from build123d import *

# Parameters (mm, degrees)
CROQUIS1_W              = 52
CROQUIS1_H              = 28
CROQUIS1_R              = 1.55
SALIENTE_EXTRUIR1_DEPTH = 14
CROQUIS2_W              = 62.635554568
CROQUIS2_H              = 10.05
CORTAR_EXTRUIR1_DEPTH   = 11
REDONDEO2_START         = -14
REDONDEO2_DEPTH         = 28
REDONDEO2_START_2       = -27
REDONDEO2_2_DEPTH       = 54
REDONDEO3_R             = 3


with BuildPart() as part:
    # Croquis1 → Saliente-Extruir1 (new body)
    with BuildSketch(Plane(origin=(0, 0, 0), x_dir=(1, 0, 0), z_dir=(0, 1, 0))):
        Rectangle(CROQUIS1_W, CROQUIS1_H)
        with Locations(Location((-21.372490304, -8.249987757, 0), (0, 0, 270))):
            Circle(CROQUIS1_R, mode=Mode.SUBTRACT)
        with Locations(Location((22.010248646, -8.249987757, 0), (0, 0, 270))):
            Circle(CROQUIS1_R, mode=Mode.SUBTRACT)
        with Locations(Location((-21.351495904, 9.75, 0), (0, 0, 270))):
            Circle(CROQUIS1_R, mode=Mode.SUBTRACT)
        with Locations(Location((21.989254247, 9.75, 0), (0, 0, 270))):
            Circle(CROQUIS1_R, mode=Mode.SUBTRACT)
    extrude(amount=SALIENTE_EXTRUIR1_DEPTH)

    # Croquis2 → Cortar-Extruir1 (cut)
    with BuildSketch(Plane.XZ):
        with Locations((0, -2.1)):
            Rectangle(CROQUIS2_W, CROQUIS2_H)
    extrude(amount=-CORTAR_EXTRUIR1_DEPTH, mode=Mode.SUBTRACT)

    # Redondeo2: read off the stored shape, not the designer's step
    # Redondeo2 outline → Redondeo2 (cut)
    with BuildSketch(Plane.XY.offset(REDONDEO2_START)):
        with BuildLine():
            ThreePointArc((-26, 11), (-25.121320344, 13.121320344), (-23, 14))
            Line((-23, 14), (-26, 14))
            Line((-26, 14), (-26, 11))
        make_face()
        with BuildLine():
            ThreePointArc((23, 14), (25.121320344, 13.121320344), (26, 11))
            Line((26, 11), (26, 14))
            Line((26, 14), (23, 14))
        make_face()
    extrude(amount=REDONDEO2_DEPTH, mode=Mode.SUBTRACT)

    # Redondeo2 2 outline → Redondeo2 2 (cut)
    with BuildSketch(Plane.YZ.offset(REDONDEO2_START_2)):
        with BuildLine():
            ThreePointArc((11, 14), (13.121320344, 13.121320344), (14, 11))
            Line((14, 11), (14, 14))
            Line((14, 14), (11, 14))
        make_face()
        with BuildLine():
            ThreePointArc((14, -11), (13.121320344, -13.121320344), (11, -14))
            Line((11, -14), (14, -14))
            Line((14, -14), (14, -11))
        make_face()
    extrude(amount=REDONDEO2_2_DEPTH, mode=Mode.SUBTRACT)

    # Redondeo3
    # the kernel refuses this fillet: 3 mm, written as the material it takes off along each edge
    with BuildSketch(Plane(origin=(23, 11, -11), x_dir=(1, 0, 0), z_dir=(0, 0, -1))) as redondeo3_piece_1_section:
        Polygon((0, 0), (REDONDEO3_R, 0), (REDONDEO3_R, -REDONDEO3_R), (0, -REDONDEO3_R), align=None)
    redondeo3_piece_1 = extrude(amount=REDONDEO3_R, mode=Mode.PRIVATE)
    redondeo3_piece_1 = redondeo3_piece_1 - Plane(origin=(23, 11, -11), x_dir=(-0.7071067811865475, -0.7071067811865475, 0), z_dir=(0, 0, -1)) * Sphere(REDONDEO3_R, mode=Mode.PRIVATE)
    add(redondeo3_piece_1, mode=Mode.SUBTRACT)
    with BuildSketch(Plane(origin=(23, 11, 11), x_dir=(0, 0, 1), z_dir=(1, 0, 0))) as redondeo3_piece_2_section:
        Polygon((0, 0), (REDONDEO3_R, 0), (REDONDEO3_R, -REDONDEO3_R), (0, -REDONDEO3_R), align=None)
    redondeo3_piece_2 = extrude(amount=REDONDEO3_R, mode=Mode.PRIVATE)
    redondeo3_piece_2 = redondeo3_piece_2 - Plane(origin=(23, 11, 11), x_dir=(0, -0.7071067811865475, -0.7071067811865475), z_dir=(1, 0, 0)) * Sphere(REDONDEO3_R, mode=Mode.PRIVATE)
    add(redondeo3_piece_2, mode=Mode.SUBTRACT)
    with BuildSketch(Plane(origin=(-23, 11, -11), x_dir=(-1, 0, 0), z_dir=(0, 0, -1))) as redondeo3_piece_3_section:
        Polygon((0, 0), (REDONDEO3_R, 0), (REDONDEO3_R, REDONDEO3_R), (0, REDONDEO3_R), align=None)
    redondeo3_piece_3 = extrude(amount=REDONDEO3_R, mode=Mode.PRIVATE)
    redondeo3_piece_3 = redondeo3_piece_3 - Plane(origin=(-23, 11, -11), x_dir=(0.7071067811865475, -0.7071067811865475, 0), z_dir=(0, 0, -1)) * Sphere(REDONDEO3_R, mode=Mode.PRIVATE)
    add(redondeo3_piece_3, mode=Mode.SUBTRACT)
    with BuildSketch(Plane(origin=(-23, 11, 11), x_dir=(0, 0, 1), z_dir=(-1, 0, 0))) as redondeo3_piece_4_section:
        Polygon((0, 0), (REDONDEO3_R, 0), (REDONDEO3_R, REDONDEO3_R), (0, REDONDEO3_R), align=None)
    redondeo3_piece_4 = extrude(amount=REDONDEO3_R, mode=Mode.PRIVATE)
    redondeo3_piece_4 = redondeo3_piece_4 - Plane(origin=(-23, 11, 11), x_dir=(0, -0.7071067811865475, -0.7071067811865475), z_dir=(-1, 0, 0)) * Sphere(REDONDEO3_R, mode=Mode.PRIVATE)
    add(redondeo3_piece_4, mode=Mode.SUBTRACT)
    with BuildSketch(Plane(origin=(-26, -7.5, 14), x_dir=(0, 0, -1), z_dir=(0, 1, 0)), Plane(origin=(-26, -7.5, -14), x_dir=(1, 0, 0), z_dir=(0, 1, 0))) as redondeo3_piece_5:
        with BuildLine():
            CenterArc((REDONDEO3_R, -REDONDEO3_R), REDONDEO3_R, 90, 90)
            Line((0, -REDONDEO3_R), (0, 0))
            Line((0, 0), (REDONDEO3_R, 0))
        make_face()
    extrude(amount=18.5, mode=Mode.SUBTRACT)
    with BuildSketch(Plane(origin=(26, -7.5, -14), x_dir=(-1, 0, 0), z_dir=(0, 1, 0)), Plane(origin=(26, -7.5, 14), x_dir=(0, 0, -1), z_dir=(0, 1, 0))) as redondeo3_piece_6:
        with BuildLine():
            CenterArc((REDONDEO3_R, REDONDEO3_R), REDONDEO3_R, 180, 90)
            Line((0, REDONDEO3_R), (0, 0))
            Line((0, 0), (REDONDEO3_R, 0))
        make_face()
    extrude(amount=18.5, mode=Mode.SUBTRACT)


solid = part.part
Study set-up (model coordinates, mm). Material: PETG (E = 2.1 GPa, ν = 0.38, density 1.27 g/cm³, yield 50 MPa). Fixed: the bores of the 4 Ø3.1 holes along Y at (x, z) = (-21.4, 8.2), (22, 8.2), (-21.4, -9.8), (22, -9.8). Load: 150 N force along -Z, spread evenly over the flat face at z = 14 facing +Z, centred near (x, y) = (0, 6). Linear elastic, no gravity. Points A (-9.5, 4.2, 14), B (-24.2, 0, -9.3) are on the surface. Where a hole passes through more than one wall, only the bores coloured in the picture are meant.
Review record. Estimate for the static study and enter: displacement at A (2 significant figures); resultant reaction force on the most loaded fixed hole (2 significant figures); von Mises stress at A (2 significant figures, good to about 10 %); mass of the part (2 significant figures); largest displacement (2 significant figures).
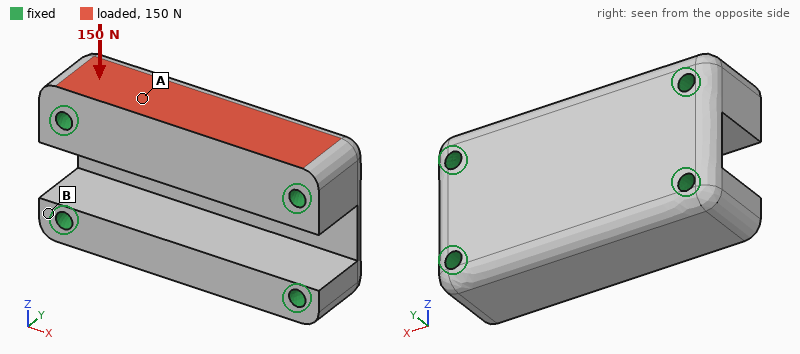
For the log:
14 µm
63 N
0.77 MPa
18 g
22 µm
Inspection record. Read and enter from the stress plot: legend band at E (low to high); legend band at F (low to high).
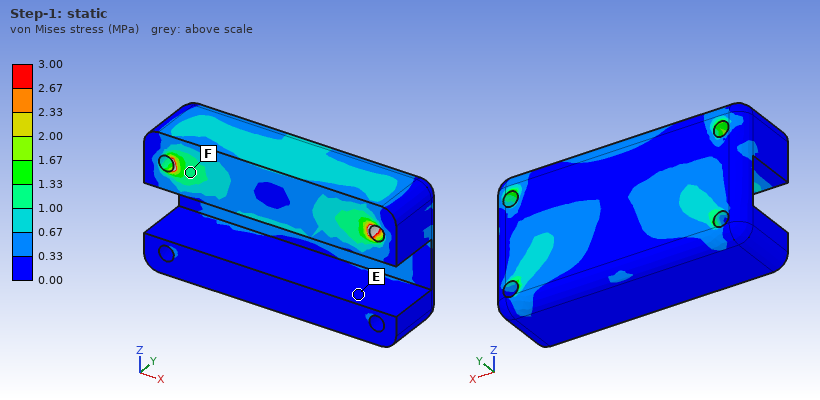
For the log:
0.00 to 0.33 MPa
1.00 to 1.33 MPa
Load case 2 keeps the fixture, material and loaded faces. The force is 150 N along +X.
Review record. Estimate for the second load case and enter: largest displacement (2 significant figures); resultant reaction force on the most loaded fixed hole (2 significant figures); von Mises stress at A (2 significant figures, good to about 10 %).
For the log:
4.3 µm
75 N
0.56 MPa
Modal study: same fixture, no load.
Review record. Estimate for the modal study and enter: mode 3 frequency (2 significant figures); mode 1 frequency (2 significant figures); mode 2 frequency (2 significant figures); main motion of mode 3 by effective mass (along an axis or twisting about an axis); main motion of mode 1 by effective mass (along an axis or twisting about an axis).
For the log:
6300 Hz
5200 Hz
5900 Hz
along Y
along Z
